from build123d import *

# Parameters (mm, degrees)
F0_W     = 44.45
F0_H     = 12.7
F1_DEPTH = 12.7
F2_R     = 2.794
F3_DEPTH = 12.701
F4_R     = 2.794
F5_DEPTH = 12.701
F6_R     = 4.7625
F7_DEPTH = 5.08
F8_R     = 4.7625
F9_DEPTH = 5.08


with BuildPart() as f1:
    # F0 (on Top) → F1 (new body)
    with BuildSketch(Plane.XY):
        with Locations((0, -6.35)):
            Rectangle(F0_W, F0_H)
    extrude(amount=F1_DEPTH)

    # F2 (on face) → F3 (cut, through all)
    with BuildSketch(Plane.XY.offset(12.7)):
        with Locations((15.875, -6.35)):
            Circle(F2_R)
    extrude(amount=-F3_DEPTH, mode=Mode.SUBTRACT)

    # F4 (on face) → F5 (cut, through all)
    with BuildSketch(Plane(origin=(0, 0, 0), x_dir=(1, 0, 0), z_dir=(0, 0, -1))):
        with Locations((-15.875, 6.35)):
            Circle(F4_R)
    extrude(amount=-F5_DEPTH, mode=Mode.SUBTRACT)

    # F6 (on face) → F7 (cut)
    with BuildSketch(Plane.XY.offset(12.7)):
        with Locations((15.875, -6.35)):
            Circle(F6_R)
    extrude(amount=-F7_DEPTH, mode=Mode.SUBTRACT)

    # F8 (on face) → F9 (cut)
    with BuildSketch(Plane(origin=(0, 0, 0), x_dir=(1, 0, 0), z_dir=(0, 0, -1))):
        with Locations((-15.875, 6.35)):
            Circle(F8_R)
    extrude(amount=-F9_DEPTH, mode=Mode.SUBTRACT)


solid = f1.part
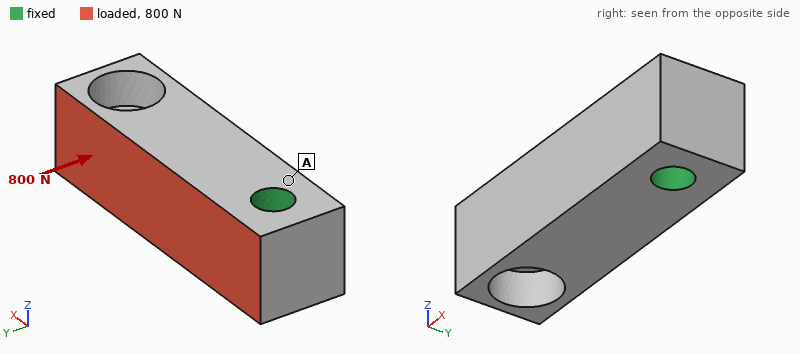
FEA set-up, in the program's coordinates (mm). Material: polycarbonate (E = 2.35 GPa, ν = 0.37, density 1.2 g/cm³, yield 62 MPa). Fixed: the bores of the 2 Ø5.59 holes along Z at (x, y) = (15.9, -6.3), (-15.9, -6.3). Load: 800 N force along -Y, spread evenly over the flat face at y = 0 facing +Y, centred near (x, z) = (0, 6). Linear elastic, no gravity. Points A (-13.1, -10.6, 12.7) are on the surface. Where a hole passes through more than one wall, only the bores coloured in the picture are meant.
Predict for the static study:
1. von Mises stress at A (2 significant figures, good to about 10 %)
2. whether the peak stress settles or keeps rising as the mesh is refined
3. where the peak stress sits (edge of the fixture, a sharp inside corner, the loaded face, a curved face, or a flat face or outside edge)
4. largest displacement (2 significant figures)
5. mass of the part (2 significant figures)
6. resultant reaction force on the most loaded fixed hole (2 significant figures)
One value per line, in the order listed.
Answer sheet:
2.1 MPa
keeps rising
edge of the fixture
50 µm
7.3 g
400 N
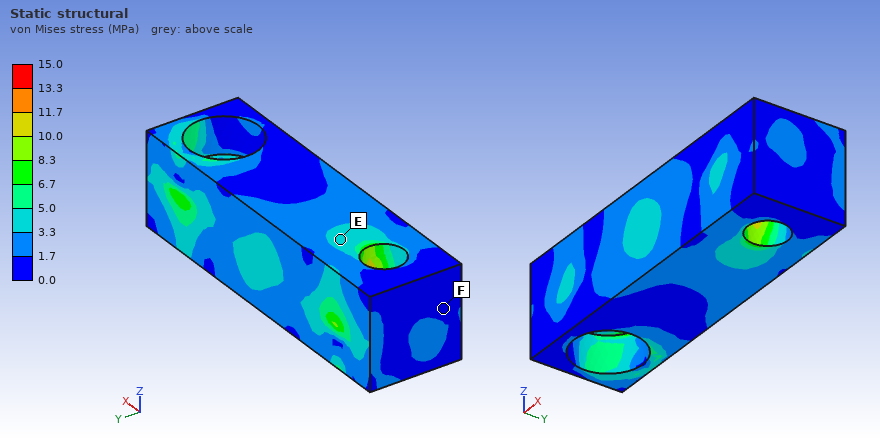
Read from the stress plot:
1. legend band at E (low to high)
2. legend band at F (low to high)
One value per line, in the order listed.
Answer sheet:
3.3 to 5.0 MPa
0.0 to 1.7 MPa
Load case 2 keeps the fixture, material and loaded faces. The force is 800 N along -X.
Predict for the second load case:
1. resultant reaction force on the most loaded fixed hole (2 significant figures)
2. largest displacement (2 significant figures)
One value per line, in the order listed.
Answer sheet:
420 N
43 µm
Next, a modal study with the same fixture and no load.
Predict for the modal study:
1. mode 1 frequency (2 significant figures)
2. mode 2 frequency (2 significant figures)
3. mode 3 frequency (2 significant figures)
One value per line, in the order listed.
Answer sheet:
8700 Hz
9100 Hz
9400 Hz
